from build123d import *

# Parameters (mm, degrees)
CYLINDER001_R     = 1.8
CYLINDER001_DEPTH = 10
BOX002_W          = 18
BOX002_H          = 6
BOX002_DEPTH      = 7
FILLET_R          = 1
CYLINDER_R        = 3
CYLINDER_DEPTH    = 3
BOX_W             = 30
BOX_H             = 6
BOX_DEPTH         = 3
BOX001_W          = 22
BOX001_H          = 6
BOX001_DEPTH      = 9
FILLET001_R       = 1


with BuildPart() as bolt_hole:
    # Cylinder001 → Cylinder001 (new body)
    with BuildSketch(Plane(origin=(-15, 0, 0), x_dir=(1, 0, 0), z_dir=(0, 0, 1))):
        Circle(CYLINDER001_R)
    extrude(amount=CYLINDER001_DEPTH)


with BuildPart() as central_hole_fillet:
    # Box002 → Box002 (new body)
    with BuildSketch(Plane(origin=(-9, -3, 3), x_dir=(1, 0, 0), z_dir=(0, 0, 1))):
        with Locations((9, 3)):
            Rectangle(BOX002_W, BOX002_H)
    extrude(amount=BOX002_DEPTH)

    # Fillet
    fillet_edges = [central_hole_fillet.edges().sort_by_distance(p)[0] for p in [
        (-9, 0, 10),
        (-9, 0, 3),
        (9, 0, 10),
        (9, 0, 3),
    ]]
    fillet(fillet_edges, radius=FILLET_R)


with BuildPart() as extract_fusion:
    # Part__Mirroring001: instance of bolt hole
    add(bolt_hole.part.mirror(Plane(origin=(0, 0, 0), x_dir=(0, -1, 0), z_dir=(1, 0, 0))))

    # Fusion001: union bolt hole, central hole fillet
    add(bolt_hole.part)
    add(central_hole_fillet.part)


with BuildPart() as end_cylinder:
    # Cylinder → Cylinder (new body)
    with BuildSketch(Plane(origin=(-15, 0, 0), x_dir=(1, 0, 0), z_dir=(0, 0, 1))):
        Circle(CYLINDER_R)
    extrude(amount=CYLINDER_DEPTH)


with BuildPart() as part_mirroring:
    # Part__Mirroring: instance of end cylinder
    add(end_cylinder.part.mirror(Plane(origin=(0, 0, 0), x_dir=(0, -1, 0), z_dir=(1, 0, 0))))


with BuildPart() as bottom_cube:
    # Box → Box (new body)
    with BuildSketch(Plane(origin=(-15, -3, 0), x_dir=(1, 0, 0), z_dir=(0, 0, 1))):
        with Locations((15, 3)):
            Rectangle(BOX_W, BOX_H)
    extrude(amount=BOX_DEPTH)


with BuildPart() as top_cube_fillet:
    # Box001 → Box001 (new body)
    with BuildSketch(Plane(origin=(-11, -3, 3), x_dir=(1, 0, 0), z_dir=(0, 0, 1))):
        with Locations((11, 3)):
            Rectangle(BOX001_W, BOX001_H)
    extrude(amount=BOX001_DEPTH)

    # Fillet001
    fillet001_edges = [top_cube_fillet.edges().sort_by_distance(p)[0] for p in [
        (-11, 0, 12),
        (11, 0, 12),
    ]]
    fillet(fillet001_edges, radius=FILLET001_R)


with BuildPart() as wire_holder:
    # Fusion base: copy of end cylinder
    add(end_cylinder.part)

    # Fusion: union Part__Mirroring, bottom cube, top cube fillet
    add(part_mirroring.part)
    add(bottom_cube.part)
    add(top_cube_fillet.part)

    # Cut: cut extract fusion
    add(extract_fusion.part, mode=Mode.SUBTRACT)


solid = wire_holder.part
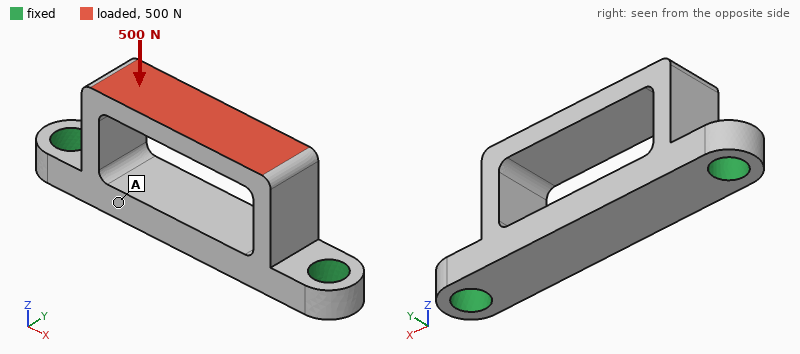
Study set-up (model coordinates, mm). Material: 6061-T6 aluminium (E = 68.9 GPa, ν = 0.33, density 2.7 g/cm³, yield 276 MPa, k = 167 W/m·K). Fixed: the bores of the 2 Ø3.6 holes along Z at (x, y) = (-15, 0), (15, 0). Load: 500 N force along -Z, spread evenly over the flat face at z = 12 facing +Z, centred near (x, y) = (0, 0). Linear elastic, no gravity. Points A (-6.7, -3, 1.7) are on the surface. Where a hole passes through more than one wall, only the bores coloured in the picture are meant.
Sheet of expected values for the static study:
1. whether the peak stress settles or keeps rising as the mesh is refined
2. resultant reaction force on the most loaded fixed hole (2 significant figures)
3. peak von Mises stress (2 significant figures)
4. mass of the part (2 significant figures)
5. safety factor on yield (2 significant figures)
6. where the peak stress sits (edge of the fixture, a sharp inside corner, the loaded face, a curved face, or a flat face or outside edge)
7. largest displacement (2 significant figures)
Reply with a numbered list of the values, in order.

1. settles
2. 270 N
3. 220 MPa
4. 2.7 g
5. 1.3
6. a curved face
7. 58 µm
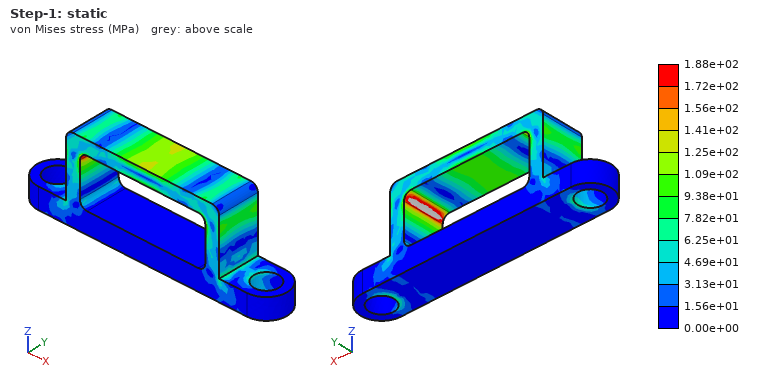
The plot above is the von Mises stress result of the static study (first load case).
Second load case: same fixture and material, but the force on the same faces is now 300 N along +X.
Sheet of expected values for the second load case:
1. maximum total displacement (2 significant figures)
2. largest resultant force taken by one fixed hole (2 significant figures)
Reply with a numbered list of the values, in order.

1. 54 µm
2. 190 N
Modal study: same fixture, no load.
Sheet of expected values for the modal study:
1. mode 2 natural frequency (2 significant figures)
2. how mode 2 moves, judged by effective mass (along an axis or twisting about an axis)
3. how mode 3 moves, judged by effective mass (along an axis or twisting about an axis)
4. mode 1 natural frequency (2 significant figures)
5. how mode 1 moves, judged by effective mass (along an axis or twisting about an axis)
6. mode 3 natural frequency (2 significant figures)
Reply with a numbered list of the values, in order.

1. 13 kHz
2. along X
3. along Z
4. 12 kHz
5. along Y
6. 21 kHz
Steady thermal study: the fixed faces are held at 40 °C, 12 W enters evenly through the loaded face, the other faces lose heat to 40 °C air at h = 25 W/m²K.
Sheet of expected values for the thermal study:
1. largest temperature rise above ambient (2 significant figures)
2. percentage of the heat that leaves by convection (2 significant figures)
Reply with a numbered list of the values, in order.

1. 43 K
2. 3.1 %
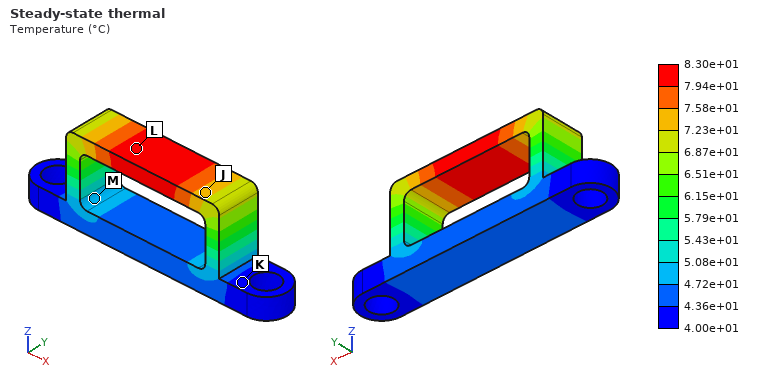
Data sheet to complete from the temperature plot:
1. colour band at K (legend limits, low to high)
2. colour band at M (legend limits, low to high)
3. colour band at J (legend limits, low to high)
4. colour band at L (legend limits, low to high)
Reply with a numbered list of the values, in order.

1. 4.00e+01 to 4.36e+01 °C
2. 4.72e+01 to 5.08e+01 °C
3. 7.23e+01 to 7.58e+01 °C
4. 7.94e+01 to 8.30e+01 °C
